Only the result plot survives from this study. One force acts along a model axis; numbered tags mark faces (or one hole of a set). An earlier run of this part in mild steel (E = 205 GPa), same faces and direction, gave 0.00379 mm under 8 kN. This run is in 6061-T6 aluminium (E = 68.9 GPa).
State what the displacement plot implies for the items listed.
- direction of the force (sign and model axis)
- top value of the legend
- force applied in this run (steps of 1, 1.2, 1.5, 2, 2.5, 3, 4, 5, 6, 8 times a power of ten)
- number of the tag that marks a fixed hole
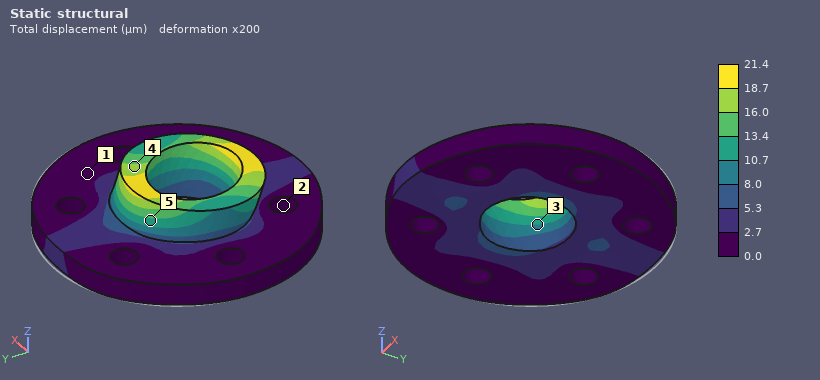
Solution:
-Y
21.4 µm
15 kN
2
